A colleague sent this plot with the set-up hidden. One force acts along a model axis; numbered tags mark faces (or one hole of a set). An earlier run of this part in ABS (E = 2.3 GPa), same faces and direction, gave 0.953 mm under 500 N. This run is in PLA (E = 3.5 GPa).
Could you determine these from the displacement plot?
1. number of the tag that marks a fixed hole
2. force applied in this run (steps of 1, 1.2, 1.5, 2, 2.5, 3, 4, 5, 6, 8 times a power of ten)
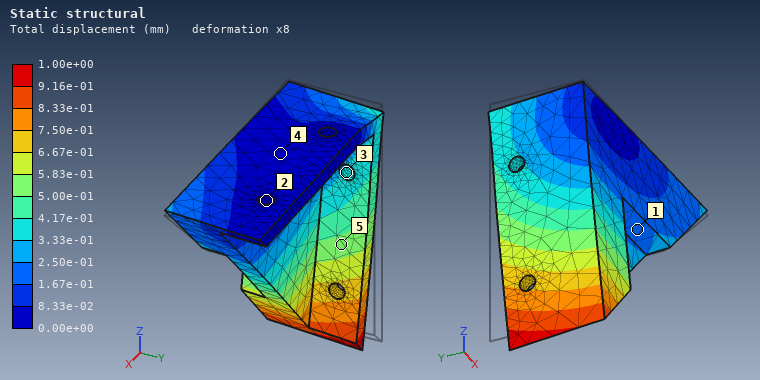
2
800 N
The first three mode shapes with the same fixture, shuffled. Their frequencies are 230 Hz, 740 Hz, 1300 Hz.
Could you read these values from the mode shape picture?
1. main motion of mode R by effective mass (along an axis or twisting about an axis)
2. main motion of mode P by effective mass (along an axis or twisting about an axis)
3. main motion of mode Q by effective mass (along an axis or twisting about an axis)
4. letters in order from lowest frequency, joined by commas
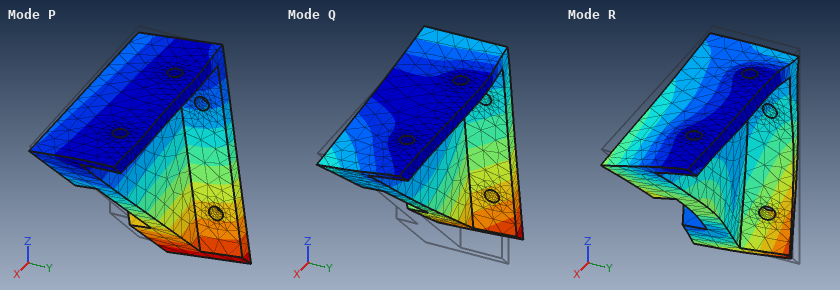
along Z
along Y
along X
P, Q, R
